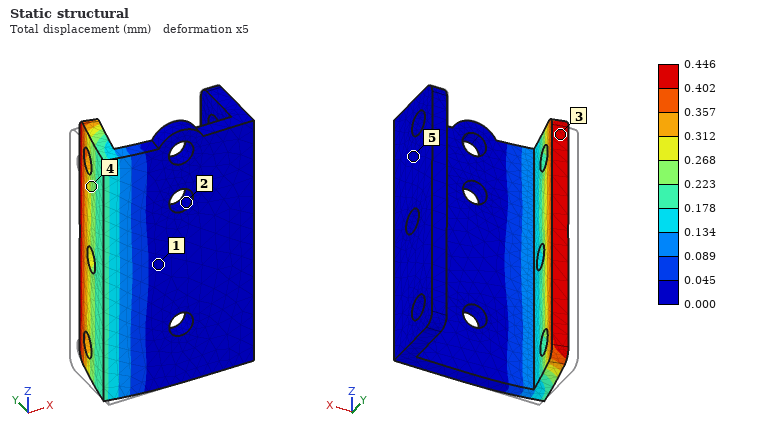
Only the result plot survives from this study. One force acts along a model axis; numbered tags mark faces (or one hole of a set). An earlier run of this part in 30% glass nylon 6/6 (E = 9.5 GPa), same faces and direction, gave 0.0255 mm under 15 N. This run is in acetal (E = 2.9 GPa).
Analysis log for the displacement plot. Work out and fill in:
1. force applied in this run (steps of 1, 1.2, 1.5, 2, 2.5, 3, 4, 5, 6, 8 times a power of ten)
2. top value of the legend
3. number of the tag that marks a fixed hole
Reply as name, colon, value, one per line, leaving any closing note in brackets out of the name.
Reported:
force applied in this run: 80 N
top value of the legend: 0.446 mm
number of the tag that marks a fixed hole: 2
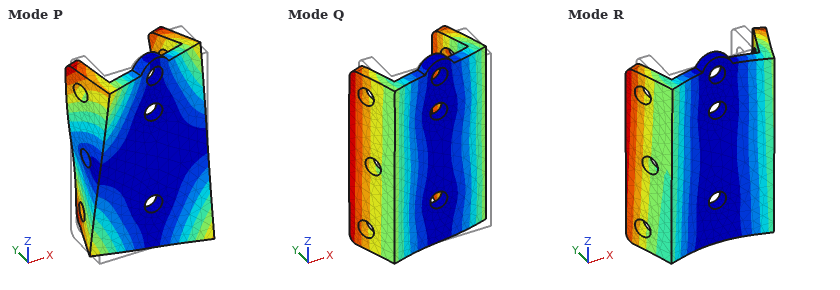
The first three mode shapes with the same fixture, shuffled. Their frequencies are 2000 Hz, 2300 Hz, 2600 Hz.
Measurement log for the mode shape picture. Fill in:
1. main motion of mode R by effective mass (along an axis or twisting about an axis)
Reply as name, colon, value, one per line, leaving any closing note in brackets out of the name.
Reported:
main motion of mode R by effective mass: along Y
